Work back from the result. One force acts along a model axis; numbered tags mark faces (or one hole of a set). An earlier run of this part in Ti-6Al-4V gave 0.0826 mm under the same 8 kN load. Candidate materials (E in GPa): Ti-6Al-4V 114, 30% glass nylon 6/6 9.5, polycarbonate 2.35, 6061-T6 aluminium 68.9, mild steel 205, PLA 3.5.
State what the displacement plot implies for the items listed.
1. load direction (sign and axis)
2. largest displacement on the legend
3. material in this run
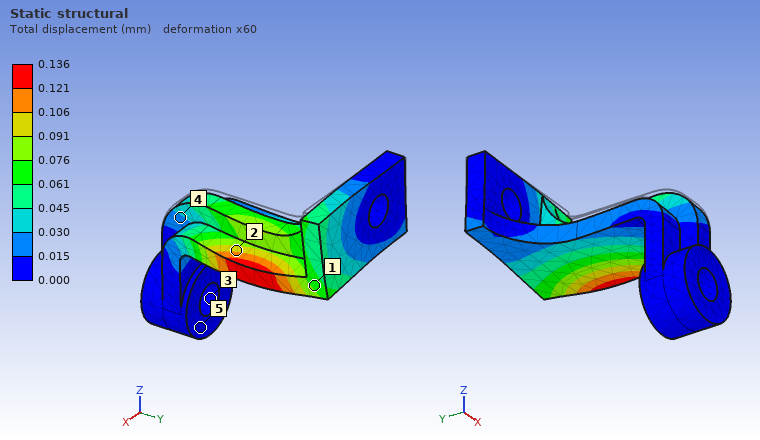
-Z
0.136 mm
6061-T6 aluminium
